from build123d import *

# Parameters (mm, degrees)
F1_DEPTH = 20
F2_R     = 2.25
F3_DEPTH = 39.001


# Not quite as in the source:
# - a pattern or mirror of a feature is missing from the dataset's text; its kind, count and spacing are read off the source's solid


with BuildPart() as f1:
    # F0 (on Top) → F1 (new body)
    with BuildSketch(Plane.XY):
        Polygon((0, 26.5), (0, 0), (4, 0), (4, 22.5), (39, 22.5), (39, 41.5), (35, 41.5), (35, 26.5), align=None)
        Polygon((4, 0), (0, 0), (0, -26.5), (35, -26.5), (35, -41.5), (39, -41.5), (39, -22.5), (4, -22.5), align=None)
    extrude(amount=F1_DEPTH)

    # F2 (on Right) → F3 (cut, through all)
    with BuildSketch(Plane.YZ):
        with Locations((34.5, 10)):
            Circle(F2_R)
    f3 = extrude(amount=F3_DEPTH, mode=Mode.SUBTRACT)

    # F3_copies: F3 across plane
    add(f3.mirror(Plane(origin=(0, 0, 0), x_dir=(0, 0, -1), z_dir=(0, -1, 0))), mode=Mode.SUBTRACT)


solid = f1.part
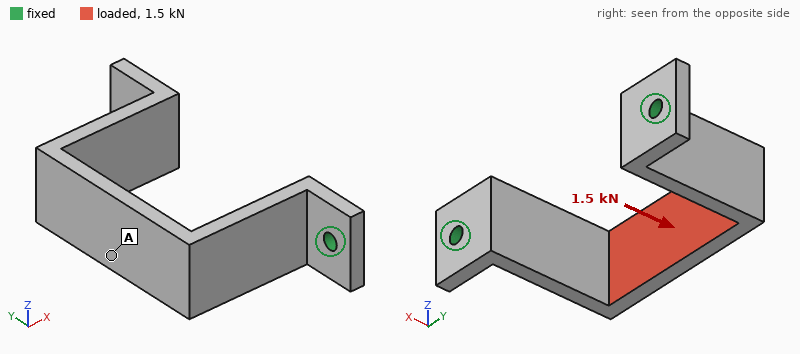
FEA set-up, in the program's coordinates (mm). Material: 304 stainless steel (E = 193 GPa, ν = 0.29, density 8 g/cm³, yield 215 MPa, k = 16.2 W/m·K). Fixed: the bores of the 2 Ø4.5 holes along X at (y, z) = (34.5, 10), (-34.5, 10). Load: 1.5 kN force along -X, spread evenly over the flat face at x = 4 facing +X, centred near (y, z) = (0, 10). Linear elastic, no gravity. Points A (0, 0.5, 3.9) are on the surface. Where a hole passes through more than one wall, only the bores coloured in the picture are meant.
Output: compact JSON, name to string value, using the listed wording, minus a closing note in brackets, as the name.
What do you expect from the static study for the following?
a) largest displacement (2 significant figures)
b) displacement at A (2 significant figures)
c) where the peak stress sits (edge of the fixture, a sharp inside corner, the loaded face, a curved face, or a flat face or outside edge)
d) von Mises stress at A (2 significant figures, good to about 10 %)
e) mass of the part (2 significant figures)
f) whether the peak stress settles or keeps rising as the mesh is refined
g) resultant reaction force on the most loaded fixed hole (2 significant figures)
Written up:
{"largest displacement": "53 µm", "displacement at A": "51 µm", "where the peak stress sits": "edge of the fixture", "von Mises stress at A": "88 MPa", "mass of the part": "97 g", "whether the peak stress settles or keeps rising as the mesh is refined": "keeps rising", "resultant reaction force on the most loaded fixed hole": "790 N"}
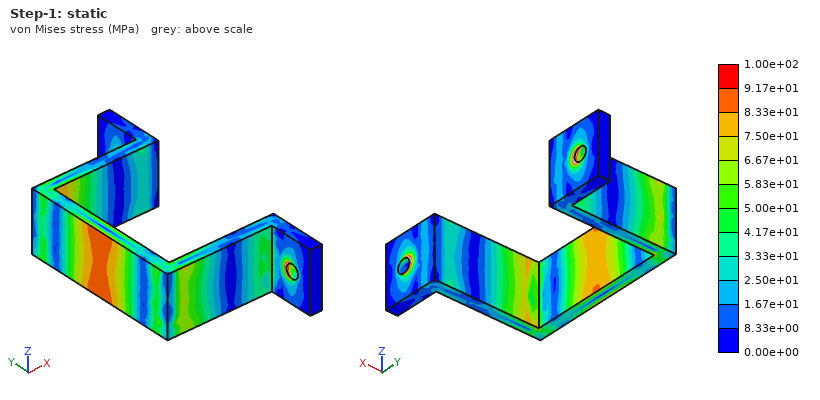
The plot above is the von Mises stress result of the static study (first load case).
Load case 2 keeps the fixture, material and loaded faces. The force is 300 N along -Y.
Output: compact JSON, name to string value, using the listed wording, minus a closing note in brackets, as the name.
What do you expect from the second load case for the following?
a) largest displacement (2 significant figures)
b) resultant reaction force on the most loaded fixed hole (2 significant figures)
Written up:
{"largest displacement": "53 µm", "resultant reaction force on the most loaded fixed hole": "180 N"}
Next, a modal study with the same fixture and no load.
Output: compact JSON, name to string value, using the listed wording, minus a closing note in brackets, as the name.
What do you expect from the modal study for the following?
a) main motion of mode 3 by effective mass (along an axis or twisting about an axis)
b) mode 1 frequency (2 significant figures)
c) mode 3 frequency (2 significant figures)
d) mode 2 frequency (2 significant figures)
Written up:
{"main motion of mode 3 by effective mass": "twisting about X", "mode 1 frequency": "1700 Hz", "mode 3 frequency": "3000 Hz", "mode 2 frequency": "1800 Hz"}
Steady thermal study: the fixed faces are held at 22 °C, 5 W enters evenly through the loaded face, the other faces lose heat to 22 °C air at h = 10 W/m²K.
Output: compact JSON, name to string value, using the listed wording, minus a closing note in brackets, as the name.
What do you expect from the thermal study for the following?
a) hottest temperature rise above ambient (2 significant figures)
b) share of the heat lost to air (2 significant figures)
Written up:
{"hottest temperature rise above ambient": "74 K", "share of the heat lost to air": "42 %"}
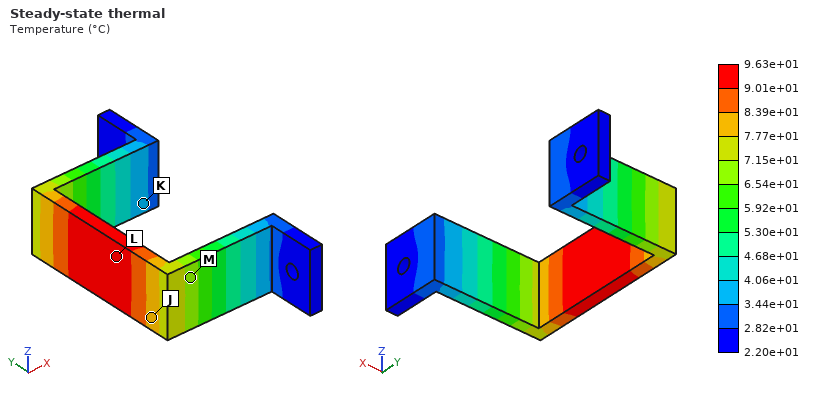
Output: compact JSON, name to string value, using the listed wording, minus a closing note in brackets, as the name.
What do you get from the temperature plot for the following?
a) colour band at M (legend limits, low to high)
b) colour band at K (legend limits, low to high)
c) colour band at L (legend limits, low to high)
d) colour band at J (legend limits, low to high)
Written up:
{"colour band at M": "6.54e+01 to 7.15e+01 °C", "colour band at K": "3.44e+01 to 4.06e+01 °C", "colour band at L": "9.01e+01 to 9.63e+01 °C", "colour band at J": "7.77e+01 to 8.39e+01 °C"}
